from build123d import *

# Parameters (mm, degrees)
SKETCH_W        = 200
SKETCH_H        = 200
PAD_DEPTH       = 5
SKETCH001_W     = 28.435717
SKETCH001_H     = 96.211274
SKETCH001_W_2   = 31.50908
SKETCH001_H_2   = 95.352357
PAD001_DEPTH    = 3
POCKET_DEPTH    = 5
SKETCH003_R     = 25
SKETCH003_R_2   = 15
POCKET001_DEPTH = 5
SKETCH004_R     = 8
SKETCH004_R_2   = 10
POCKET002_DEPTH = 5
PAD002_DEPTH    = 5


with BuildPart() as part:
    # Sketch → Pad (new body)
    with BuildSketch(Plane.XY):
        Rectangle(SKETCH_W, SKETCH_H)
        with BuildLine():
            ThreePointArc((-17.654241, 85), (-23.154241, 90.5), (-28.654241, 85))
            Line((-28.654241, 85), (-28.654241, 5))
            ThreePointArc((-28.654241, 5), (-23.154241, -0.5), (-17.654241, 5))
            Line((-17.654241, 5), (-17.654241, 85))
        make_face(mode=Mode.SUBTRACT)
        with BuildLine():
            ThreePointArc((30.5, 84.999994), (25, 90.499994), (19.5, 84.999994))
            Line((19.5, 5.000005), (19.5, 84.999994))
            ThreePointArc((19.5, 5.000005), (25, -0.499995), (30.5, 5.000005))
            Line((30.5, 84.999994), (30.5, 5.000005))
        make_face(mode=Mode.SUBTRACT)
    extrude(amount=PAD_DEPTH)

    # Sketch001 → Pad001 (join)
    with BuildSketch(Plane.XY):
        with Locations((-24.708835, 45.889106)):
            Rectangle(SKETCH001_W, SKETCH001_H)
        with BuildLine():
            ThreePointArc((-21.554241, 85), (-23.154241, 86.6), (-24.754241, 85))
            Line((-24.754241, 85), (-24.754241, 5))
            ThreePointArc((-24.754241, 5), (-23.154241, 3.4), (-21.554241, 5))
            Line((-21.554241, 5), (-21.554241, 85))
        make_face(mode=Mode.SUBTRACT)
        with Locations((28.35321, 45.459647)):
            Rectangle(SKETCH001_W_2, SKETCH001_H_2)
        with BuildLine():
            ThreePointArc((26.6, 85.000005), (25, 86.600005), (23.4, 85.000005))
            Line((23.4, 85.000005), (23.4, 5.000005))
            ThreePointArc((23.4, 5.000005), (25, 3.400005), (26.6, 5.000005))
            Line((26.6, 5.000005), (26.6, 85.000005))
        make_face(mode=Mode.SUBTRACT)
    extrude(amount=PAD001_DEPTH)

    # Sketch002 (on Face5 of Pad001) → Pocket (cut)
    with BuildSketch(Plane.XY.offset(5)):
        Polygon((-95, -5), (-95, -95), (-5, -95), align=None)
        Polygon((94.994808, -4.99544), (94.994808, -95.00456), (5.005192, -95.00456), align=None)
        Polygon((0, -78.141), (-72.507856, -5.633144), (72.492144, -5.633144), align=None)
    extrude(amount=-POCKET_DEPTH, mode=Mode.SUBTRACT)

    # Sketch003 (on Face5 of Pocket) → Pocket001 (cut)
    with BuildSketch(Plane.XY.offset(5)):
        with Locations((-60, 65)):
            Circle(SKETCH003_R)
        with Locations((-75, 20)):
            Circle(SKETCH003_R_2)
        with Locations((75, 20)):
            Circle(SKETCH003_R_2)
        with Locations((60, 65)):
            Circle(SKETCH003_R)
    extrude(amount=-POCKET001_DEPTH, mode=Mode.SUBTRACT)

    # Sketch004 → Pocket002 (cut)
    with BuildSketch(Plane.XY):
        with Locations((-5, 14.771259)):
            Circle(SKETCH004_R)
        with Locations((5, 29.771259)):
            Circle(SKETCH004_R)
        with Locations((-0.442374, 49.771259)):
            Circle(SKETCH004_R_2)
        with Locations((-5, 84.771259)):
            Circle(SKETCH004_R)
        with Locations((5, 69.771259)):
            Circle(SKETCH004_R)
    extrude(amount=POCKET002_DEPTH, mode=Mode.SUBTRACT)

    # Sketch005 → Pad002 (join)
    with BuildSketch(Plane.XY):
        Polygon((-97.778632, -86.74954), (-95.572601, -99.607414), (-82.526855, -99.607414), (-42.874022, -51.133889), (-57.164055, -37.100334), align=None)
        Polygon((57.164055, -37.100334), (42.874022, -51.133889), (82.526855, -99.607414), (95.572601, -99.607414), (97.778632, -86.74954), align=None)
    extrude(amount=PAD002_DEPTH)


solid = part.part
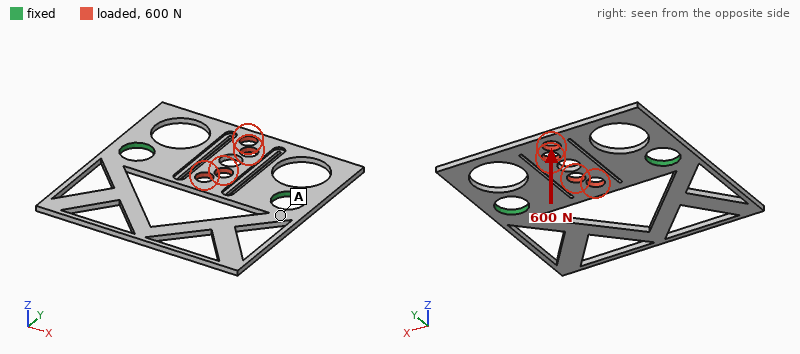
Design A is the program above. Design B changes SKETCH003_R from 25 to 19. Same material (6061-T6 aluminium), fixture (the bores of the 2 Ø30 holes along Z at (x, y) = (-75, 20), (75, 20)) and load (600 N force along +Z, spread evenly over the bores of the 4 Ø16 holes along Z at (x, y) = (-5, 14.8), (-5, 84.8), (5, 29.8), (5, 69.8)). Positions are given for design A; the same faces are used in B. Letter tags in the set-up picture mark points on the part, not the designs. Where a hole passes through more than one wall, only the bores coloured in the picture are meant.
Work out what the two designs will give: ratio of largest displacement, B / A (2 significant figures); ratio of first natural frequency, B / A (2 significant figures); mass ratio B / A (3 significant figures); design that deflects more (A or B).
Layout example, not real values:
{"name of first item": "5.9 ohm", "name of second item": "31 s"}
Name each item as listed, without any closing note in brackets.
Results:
{"ratio of largest displacement, B / A": "0.74", "ratio of first natural frequency, B / A": "1.00", "mass ratio B / A": "1.08", "design that deflects more": "A"}
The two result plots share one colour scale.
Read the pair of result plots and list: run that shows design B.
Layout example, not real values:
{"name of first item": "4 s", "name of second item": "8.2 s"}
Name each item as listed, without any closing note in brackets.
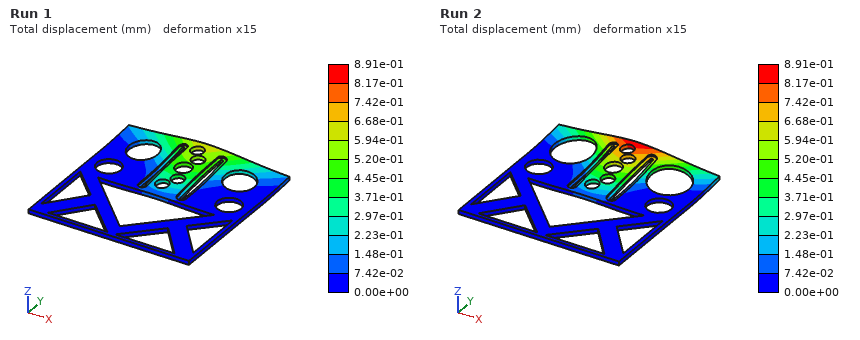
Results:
{"run that shows design B": "Run 1"}
